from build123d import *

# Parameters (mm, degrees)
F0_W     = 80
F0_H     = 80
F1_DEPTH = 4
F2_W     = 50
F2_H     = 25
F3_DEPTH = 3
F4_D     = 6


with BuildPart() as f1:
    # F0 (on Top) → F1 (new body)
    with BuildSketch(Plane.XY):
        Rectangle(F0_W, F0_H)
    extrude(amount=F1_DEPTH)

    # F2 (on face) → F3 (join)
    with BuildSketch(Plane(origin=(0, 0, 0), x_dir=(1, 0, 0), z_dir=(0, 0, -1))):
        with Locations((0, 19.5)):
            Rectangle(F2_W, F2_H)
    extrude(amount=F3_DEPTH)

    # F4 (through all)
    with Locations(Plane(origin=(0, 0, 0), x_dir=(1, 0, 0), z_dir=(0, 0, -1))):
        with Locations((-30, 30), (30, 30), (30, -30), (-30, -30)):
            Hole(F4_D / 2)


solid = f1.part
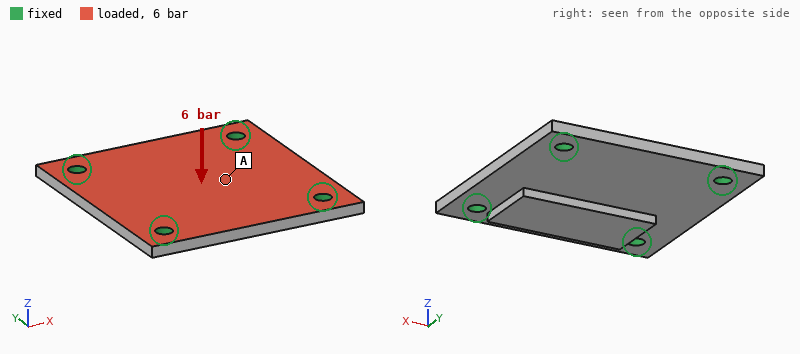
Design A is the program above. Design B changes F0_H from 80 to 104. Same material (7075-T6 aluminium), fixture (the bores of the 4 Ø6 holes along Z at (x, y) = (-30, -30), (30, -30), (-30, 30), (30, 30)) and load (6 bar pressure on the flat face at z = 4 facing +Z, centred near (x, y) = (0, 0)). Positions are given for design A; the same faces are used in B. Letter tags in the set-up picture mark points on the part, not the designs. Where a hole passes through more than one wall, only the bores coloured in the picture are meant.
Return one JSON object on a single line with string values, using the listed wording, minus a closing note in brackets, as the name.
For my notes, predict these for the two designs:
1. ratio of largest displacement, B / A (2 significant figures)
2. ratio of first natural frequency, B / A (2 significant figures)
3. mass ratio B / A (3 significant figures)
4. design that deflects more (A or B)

{"ratio of largest displacement, B / A": "1.1", "ratio of first natural frequency, B / A": "1.0", "mass ratio B / A": "1.27", "design that deflects more": "B"}
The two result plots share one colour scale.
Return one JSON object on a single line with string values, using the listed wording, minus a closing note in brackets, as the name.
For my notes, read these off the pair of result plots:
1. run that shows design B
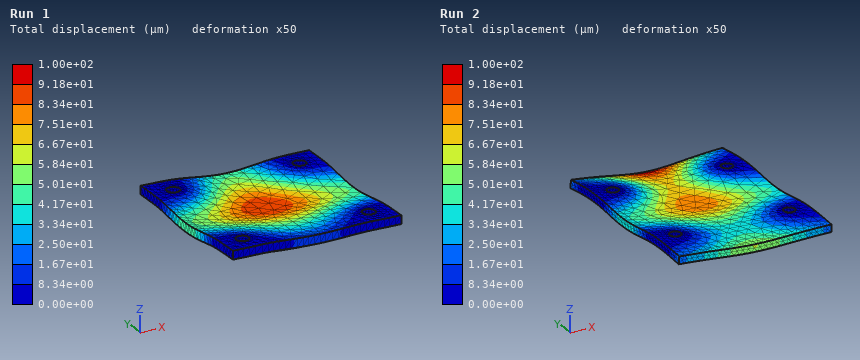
{"run that shows design B": "Run 2"}
